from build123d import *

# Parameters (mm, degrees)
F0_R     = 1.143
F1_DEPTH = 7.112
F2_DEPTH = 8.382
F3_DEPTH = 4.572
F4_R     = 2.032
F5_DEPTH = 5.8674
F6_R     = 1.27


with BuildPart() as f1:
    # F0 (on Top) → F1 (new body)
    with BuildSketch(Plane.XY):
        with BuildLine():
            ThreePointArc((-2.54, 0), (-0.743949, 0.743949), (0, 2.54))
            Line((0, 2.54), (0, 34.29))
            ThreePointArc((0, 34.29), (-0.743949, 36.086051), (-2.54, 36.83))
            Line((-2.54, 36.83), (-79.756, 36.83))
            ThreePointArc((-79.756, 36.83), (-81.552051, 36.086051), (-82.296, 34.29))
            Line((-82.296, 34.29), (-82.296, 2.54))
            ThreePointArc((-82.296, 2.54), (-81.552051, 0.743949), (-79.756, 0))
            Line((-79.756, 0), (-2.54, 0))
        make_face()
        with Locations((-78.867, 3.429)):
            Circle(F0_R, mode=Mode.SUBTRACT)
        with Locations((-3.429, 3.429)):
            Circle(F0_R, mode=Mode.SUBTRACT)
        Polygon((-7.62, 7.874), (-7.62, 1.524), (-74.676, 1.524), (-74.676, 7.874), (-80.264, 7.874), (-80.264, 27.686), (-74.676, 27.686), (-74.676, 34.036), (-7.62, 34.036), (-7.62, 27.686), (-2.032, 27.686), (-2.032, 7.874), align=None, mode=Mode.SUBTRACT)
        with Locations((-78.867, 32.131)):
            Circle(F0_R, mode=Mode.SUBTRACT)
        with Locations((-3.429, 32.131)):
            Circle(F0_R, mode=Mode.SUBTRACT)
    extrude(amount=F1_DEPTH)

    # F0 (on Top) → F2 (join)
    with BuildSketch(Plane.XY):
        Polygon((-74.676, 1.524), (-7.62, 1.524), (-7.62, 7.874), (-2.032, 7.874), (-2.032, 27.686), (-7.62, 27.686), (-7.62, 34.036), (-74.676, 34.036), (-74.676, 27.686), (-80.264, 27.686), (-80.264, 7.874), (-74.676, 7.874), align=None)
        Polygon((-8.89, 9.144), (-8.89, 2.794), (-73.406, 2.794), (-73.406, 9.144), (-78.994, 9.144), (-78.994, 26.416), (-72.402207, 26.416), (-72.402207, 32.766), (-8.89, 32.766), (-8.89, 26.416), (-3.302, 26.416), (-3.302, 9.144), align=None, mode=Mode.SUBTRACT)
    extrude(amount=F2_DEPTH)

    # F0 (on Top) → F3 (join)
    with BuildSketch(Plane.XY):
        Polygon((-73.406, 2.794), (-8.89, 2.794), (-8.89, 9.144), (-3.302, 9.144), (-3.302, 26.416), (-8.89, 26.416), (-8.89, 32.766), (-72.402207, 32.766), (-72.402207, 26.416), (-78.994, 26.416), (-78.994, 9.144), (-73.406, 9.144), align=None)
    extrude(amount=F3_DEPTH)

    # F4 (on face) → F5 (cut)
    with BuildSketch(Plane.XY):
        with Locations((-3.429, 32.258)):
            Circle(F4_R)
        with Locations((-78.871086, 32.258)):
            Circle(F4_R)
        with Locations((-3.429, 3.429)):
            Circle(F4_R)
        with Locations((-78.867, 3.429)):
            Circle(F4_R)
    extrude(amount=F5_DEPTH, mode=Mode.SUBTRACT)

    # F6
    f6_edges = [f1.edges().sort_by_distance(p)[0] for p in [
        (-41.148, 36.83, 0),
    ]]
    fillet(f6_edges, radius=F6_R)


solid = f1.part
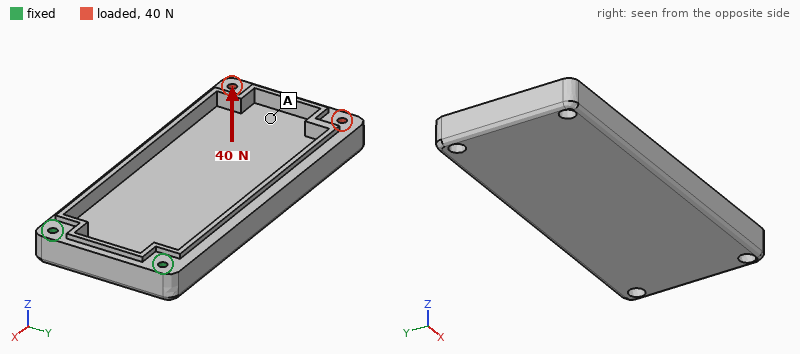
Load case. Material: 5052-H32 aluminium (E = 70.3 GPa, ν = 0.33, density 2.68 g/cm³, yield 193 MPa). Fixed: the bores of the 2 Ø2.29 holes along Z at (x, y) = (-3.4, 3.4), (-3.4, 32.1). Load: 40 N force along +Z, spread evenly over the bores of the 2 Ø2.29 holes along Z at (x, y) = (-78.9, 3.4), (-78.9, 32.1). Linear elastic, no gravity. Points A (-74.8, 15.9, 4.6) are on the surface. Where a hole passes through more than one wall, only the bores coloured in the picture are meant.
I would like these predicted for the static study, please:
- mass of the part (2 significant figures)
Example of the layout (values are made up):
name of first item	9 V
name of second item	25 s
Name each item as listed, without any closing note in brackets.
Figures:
mass of the part	43 g
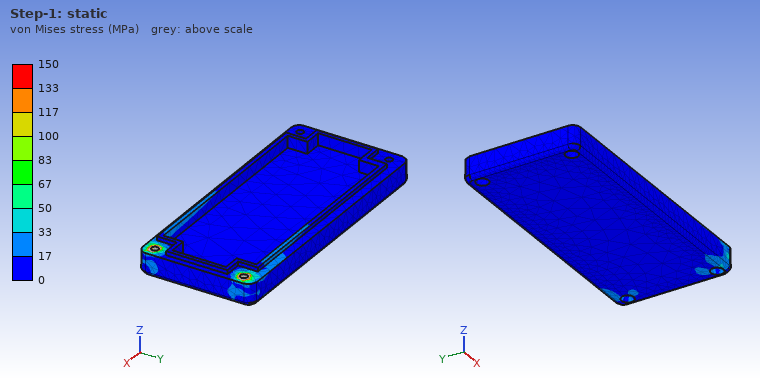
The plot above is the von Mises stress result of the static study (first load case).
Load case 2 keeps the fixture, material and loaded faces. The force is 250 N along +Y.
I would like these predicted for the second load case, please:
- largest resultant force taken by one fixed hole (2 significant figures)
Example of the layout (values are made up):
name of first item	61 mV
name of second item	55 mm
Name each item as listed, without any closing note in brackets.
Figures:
largest resultant force taken by one fixed hole	650 N
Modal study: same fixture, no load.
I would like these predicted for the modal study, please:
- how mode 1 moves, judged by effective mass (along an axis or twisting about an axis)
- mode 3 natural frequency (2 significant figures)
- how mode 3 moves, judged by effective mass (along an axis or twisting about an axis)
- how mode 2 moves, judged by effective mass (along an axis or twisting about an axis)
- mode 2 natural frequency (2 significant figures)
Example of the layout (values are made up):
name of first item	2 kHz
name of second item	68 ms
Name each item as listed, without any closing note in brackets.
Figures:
how mode 1 moves, judged by effective mass	along Z
mode 3 natural frequency	3300 Hz
how mode 3 moves, judged by effective mass	along Y
how mode 2 moves, judged by effective mass	along Y
mode 2 natural frequency	2100 Hz
